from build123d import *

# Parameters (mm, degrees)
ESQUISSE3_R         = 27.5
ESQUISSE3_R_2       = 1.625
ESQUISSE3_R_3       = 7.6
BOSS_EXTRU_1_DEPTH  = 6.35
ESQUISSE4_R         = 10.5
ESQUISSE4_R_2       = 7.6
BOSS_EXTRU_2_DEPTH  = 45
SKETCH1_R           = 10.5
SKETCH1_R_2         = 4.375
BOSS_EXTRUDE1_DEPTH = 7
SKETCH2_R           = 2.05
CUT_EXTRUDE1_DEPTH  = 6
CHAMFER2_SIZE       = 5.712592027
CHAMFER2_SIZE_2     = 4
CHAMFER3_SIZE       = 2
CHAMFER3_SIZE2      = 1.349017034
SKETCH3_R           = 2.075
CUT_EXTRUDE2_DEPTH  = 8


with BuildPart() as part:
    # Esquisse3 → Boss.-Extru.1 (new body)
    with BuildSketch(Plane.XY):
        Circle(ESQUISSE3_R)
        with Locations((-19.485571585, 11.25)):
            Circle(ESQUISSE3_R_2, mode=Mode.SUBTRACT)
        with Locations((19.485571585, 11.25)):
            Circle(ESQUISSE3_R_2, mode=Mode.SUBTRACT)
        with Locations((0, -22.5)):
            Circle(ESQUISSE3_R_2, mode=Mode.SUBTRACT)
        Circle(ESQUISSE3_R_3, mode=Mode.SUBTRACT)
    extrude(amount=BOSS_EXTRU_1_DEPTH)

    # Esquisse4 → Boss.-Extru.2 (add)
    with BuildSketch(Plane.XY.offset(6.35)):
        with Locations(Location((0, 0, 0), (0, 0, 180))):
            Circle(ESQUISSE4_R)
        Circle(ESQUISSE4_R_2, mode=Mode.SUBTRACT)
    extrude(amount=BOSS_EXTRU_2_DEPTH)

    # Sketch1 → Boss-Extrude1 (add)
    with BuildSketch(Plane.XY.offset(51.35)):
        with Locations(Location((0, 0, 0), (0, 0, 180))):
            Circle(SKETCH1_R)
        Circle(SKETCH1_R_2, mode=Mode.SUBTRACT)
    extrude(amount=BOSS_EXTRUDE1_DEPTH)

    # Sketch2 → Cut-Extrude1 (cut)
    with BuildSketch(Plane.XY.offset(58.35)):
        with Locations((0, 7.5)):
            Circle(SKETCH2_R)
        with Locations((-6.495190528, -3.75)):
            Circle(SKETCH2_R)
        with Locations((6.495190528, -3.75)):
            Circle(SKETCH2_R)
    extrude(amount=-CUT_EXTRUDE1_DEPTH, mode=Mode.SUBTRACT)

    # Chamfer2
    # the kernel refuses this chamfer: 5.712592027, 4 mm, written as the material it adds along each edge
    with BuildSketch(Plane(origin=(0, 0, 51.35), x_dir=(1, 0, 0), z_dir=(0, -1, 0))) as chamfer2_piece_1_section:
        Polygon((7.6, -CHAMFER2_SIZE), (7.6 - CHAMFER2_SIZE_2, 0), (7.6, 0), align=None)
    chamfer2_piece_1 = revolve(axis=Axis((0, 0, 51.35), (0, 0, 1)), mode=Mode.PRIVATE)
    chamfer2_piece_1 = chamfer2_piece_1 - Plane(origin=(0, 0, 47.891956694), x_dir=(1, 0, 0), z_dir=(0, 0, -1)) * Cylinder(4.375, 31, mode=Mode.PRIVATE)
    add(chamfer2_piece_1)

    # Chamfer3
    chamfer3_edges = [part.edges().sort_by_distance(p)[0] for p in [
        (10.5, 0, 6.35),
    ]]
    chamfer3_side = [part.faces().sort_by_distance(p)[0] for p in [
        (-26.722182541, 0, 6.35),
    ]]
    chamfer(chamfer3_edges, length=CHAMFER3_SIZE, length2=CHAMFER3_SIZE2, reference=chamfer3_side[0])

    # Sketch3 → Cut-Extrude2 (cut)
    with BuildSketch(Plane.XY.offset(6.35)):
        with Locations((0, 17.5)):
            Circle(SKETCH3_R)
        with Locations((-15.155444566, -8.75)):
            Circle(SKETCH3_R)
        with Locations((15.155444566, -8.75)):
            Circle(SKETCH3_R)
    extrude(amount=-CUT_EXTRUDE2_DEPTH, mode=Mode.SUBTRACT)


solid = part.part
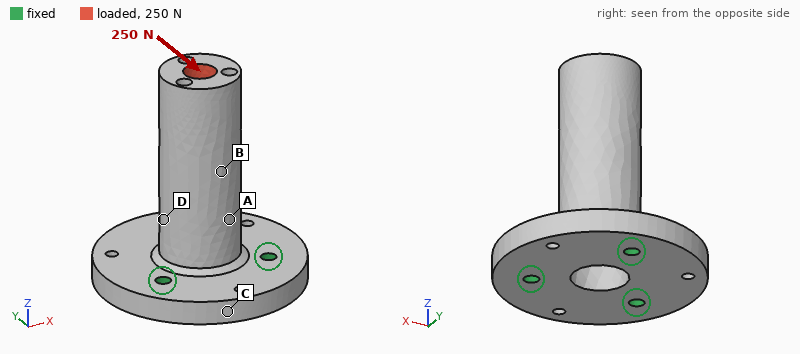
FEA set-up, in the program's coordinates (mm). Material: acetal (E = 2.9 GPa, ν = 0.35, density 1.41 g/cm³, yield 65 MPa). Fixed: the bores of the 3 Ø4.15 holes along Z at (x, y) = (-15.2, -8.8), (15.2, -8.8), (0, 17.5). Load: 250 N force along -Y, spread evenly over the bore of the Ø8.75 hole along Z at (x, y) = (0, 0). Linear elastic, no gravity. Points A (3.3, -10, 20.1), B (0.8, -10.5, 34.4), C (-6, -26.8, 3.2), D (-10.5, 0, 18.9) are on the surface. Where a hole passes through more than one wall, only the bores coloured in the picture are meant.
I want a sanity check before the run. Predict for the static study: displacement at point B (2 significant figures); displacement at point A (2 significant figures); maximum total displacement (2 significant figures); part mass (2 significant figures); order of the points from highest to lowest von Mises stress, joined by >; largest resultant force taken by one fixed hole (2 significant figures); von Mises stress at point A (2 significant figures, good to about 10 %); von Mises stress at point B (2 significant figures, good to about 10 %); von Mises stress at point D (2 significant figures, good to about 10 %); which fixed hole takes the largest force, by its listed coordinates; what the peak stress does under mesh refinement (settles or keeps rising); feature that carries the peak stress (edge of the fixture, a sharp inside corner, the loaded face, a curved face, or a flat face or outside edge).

0.50 mm
0.24 mm
1.0 mm
33 g
A > B > D > C
500 N
12 MPa
7.8 MPa
4.6 MPa
(0, 17.5)
keeps rising
edge of the fixture
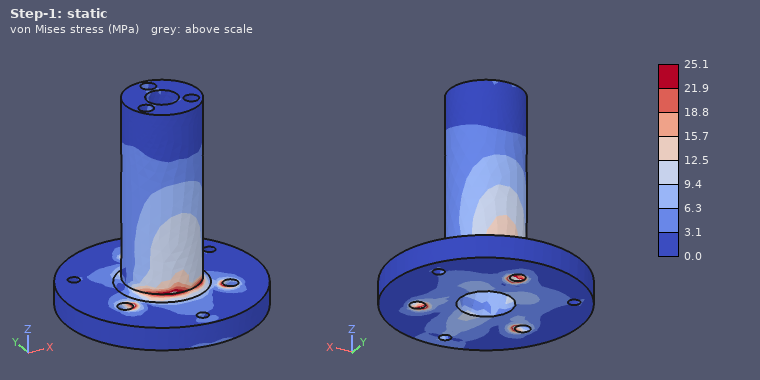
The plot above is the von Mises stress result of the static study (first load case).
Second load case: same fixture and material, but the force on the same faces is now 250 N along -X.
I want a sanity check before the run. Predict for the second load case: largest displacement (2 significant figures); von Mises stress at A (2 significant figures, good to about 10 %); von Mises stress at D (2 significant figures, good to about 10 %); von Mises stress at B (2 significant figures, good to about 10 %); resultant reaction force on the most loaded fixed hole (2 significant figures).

1.0 mm
6.1 MPa
13 MPa
4.4 MPa
440 N
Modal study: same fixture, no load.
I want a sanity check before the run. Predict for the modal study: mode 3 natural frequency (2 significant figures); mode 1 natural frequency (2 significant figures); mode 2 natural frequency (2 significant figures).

3900 Hz
1100 Hz
1100 Hz
